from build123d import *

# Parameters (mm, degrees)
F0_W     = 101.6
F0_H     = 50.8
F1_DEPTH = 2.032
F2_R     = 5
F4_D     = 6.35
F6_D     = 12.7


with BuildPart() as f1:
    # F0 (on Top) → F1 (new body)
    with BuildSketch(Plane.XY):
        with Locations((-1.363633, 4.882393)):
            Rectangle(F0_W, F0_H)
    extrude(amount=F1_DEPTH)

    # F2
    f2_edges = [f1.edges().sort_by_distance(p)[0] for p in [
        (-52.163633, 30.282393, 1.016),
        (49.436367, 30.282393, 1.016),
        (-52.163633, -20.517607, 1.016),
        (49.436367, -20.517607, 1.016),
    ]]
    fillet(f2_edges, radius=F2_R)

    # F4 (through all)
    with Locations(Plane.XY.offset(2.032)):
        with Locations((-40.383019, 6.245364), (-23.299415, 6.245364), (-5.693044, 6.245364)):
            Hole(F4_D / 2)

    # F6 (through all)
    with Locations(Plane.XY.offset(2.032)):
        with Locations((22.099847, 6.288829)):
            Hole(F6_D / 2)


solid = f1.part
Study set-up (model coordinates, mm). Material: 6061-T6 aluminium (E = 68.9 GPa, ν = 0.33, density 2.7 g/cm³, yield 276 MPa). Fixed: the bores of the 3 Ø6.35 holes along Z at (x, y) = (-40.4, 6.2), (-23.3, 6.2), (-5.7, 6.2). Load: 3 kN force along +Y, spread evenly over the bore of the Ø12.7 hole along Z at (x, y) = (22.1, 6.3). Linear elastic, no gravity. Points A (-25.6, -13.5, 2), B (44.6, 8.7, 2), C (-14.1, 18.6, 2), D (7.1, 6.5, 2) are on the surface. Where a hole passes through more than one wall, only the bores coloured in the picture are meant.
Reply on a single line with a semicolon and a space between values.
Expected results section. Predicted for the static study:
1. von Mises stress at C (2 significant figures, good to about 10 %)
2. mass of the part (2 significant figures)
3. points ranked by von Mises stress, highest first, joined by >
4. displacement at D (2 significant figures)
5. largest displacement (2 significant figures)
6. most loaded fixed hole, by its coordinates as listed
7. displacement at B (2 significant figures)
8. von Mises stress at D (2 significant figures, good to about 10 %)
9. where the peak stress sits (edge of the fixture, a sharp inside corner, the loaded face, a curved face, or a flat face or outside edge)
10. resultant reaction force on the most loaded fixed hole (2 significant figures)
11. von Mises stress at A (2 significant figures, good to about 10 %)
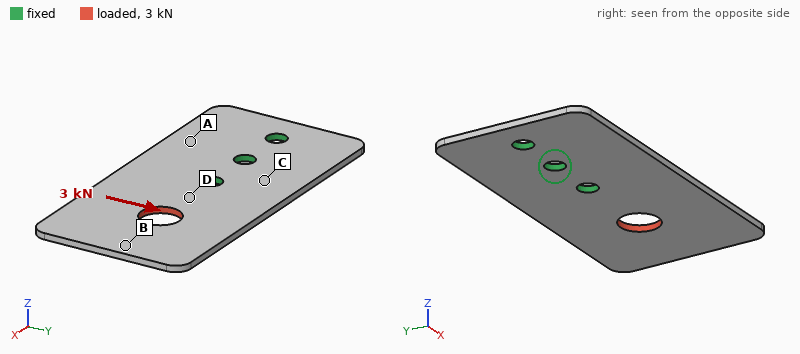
55 MPa; 27 g; D > C > A > B; 0.045 mm; 0.18 mm; (-5.7, 6.2); 0.16 mm; 81 MPa; edge of the fixture; 5.0 kN; 39 MPa
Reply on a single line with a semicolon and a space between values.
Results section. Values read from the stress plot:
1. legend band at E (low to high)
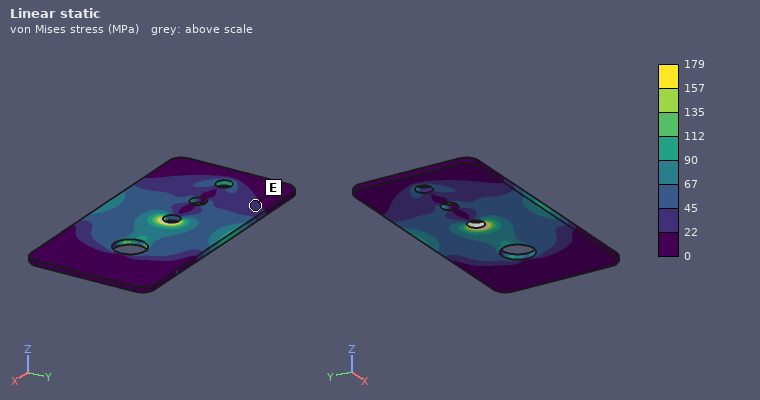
22 to 45 MPa
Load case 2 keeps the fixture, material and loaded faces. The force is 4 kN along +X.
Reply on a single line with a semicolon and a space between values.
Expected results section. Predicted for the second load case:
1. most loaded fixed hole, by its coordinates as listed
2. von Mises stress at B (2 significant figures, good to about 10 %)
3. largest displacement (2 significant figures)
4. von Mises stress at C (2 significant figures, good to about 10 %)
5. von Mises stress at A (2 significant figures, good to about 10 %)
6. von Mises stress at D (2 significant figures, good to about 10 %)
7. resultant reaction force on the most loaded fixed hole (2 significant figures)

(-5.7, 6.2); 19 MPa; 37 µm; 24 MPa; 12 MPa; 72 MPa; 2.7 kN
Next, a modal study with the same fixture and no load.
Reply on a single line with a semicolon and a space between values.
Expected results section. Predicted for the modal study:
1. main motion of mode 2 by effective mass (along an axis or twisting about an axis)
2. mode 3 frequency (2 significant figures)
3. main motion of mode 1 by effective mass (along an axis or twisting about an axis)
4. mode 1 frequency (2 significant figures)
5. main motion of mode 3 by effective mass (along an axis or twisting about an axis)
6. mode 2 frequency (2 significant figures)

twisting about X; 2600 Hz; along Z; 540 Hz; along Z; 1100 Hz
